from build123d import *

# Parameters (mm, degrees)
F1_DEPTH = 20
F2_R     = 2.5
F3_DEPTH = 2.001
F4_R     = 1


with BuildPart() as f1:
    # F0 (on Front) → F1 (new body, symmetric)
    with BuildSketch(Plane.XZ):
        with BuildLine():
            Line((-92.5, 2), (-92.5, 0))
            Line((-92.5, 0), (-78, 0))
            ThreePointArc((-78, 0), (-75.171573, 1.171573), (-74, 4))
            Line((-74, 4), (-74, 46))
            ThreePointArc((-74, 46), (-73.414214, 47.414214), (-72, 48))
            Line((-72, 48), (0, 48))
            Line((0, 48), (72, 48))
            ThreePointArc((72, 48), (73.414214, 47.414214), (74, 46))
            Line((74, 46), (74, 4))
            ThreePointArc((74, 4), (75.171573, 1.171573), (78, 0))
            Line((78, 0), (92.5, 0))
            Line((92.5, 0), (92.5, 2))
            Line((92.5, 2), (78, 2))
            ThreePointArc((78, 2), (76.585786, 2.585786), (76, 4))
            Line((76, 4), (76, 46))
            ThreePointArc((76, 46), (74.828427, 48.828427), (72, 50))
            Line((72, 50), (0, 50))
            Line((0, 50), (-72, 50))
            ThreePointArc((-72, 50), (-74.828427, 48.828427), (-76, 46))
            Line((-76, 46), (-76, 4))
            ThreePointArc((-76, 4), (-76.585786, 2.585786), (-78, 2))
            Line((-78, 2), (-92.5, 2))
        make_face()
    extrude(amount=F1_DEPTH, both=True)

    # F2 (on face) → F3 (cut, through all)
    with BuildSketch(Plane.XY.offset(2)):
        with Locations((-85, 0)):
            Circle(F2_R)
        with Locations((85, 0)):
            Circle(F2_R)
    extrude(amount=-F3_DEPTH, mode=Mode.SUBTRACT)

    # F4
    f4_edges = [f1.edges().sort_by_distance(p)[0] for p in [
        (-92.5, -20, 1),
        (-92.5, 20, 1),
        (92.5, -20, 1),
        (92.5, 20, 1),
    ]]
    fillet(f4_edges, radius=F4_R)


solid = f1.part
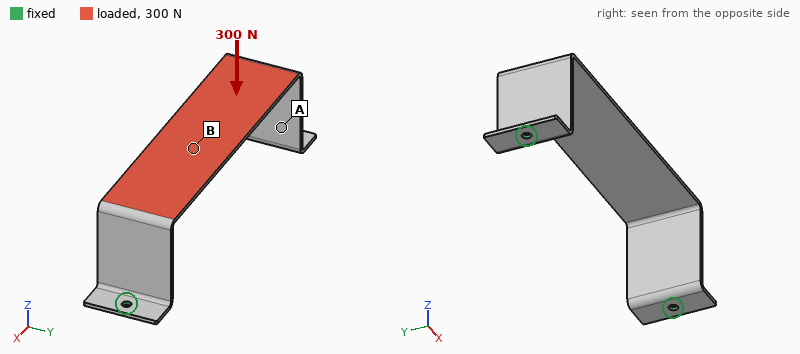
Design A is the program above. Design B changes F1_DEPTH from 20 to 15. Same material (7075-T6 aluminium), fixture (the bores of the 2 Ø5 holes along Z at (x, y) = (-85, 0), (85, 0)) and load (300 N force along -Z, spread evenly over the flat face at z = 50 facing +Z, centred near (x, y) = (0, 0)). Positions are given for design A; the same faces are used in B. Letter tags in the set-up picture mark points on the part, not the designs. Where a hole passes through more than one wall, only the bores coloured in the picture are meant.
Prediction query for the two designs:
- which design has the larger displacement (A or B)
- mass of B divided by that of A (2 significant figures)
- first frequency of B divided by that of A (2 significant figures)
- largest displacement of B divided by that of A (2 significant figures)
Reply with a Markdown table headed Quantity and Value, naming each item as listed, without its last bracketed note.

| Quantity | Value |
|---|---|
| which design has the larger displacement | B |
| mass of B divided by that of A | 0.75 |
| first frequency of B divided by that of A | 1.0 |
| largest displacement of B divided by that of A | 1.3 |
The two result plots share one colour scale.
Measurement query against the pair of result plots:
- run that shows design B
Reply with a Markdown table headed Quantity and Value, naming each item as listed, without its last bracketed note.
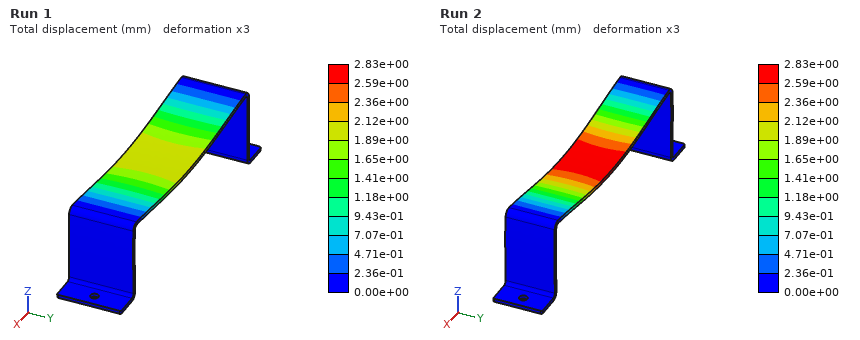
| Quantity | Value |
|---|---|
| run that shows design B | Run 2 |
